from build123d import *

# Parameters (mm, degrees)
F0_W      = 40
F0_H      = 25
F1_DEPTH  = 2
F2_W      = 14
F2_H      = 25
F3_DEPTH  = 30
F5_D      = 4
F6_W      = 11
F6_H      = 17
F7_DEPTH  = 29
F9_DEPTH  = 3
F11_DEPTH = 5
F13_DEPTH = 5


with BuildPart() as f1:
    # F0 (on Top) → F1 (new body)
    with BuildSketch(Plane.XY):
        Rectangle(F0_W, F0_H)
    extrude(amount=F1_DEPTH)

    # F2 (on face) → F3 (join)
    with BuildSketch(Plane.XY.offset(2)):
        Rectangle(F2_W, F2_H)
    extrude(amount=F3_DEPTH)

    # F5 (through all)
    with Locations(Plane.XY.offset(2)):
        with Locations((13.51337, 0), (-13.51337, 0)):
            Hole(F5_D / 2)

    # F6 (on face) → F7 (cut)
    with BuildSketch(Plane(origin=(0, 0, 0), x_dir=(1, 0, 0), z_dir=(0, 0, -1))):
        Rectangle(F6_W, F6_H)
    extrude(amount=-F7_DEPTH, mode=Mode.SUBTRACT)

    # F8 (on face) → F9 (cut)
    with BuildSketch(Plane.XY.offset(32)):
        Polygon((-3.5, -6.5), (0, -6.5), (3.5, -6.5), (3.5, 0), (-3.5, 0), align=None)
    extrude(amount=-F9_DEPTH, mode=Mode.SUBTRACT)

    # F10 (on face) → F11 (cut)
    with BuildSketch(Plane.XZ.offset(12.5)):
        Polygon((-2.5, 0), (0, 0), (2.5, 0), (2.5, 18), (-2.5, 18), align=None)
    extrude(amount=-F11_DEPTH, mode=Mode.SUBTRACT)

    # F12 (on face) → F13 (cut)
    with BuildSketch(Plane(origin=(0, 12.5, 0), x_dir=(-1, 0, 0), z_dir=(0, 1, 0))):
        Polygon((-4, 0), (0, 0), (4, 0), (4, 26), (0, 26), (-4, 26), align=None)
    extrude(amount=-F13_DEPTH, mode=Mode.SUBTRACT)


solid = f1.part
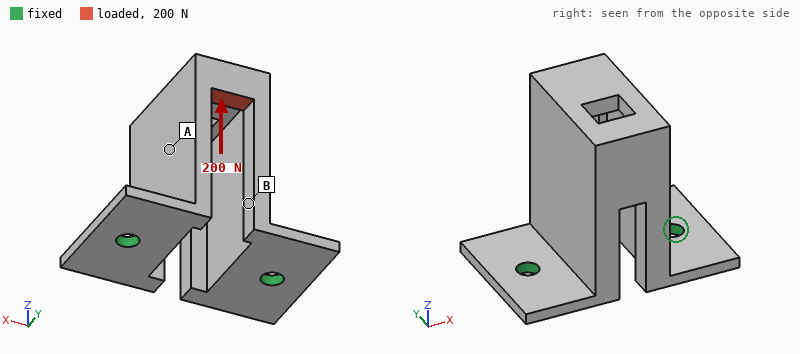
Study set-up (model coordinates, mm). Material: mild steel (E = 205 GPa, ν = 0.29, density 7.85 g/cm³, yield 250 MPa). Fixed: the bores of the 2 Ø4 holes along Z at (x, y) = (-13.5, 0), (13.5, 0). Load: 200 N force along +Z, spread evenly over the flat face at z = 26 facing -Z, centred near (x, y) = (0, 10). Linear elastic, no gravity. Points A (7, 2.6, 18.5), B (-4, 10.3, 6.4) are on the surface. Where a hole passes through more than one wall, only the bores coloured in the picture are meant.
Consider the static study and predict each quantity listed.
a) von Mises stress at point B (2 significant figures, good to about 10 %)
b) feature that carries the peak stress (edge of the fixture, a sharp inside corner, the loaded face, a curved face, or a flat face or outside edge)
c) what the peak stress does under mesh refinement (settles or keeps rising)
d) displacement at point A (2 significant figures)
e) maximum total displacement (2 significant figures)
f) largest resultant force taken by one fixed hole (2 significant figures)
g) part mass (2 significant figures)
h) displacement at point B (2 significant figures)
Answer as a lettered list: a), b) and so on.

a) 19 MPa
b) edge of the fixture
c) keeps rising
d) 21 µm
e) 39 µm
f) 100 N
g) 45 g
h) 16 µm
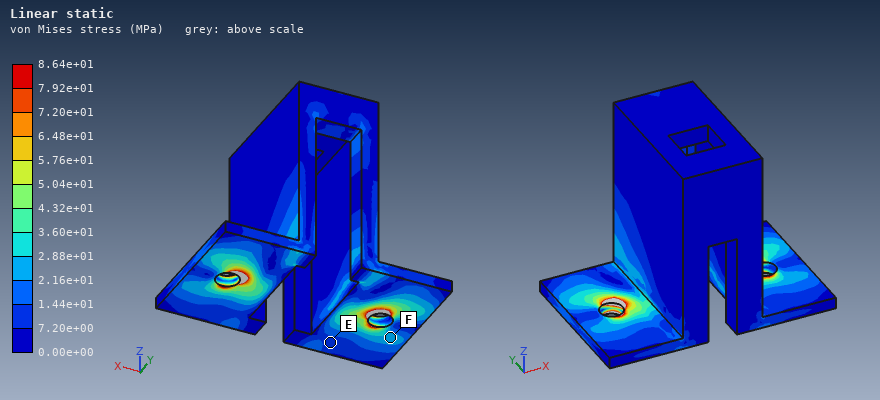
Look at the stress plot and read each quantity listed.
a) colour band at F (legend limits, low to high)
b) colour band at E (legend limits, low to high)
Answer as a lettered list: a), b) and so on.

a) 2.16e+01 to 2.88e+01 MPa
b) 7.20e+00 to 1.44e+01 MPa
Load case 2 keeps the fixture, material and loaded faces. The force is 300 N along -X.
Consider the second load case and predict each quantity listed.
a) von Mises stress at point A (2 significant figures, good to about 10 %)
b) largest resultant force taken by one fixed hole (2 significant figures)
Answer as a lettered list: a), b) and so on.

a) 34 MPa
b) 390 N
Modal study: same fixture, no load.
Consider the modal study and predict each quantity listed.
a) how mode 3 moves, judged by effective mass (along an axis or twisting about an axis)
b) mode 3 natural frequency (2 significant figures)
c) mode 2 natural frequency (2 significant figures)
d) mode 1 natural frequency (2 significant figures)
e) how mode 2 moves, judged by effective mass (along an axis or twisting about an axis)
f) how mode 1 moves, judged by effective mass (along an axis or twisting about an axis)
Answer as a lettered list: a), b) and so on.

a) twisting about Z
b) 5700 Hz
c) 2800 Hz
d) 1700 Hz
e) along X
f) along Y
